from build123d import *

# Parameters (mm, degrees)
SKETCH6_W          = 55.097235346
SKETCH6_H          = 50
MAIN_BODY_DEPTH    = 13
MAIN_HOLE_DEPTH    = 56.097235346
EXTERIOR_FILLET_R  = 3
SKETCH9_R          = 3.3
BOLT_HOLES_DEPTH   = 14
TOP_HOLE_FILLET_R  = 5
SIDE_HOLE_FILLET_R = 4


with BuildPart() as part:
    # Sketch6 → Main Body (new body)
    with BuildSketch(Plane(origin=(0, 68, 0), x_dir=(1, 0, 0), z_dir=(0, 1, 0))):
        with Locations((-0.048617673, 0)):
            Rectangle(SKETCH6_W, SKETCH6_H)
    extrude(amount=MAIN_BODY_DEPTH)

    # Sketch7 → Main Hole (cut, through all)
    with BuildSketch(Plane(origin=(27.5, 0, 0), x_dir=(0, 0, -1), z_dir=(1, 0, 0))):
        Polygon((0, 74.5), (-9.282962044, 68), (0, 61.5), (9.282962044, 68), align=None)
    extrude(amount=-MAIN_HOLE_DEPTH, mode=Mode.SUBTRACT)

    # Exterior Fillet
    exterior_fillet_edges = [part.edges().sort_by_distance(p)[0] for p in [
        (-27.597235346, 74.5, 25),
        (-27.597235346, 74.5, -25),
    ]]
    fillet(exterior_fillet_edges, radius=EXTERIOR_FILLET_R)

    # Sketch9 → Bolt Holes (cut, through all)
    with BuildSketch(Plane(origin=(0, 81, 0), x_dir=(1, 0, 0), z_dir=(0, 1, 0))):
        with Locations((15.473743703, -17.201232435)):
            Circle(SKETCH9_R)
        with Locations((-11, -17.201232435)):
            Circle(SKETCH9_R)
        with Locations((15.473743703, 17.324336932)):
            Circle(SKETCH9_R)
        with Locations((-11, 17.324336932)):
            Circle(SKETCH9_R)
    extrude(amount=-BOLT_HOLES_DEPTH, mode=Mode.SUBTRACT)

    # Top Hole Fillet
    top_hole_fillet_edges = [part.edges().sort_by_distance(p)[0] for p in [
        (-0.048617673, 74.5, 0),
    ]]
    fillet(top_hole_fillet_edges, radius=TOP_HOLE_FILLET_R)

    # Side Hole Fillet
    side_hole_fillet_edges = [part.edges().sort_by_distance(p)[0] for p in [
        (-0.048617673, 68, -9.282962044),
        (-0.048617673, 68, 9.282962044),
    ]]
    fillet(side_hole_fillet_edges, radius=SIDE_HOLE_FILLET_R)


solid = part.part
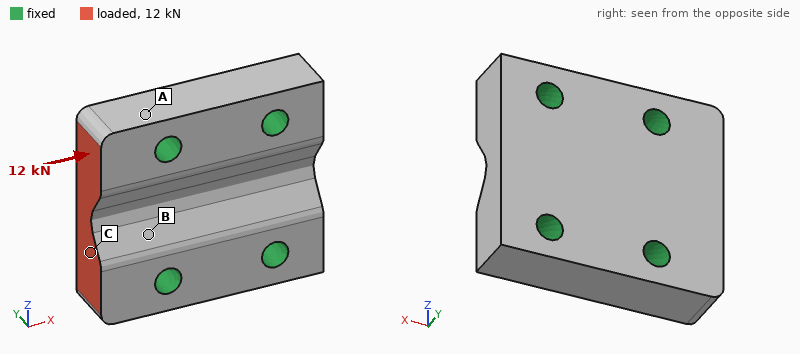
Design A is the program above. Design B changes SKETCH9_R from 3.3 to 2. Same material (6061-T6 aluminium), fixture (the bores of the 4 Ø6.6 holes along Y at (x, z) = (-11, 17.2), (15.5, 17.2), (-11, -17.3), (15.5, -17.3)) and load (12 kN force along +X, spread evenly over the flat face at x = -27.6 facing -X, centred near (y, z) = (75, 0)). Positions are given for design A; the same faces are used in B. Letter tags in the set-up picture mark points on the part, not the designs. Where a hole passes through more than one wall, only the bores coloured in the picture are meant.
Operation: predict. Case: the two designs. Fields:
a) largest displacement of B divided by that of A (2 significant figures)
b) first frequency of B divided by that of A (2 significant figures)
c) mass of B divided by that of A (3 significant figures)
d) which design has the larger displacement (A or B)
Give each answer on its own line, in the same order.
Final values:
1.1
0.84
1.04
B
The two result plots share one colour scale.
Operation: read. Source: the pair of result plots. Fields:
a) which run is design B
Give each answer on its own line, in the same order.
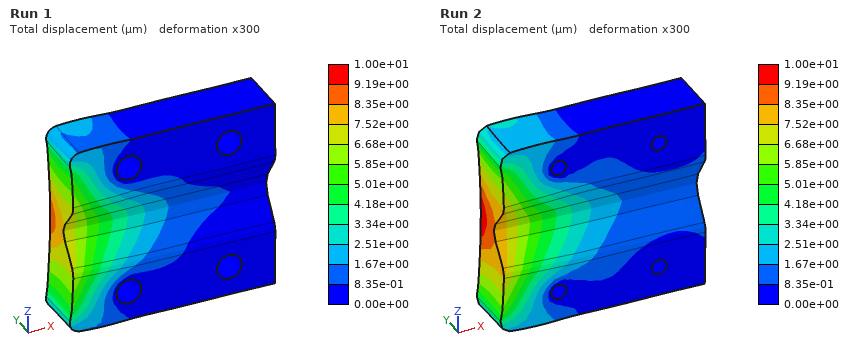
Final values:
Run 2
